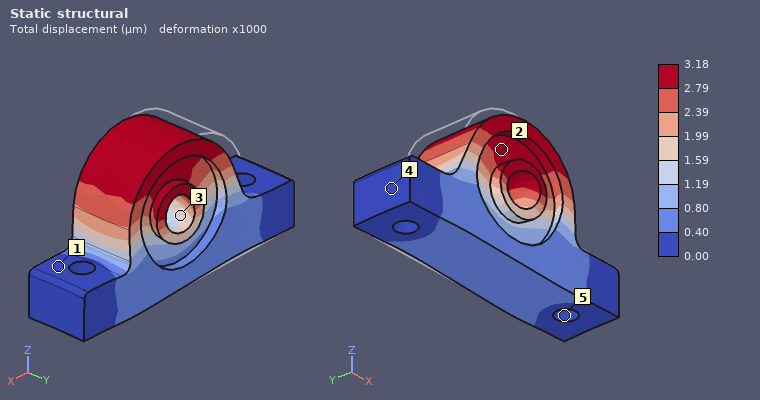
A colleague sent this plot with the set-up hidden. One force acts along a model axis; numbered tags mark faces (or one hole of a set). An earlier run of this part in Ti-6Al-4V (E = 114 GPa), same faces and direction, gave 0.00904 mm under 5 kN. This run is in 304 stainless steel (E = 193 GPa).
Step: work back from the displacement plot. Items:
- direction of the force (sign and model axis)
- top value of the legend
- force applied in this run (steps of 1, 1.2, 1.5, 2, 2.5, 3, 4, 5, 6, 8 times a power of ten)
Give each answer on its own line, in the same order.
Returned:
+X
3.18 µm
3 kN
